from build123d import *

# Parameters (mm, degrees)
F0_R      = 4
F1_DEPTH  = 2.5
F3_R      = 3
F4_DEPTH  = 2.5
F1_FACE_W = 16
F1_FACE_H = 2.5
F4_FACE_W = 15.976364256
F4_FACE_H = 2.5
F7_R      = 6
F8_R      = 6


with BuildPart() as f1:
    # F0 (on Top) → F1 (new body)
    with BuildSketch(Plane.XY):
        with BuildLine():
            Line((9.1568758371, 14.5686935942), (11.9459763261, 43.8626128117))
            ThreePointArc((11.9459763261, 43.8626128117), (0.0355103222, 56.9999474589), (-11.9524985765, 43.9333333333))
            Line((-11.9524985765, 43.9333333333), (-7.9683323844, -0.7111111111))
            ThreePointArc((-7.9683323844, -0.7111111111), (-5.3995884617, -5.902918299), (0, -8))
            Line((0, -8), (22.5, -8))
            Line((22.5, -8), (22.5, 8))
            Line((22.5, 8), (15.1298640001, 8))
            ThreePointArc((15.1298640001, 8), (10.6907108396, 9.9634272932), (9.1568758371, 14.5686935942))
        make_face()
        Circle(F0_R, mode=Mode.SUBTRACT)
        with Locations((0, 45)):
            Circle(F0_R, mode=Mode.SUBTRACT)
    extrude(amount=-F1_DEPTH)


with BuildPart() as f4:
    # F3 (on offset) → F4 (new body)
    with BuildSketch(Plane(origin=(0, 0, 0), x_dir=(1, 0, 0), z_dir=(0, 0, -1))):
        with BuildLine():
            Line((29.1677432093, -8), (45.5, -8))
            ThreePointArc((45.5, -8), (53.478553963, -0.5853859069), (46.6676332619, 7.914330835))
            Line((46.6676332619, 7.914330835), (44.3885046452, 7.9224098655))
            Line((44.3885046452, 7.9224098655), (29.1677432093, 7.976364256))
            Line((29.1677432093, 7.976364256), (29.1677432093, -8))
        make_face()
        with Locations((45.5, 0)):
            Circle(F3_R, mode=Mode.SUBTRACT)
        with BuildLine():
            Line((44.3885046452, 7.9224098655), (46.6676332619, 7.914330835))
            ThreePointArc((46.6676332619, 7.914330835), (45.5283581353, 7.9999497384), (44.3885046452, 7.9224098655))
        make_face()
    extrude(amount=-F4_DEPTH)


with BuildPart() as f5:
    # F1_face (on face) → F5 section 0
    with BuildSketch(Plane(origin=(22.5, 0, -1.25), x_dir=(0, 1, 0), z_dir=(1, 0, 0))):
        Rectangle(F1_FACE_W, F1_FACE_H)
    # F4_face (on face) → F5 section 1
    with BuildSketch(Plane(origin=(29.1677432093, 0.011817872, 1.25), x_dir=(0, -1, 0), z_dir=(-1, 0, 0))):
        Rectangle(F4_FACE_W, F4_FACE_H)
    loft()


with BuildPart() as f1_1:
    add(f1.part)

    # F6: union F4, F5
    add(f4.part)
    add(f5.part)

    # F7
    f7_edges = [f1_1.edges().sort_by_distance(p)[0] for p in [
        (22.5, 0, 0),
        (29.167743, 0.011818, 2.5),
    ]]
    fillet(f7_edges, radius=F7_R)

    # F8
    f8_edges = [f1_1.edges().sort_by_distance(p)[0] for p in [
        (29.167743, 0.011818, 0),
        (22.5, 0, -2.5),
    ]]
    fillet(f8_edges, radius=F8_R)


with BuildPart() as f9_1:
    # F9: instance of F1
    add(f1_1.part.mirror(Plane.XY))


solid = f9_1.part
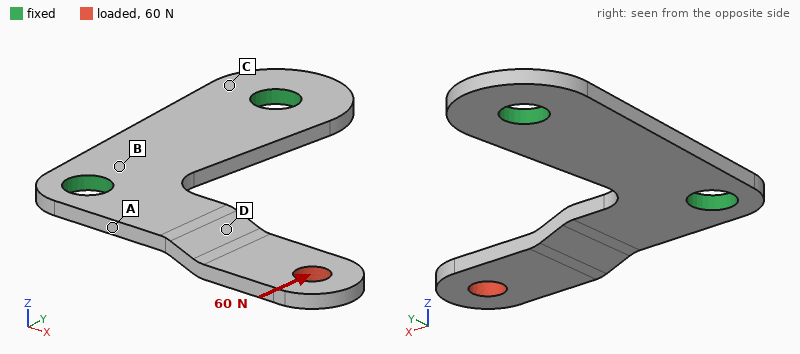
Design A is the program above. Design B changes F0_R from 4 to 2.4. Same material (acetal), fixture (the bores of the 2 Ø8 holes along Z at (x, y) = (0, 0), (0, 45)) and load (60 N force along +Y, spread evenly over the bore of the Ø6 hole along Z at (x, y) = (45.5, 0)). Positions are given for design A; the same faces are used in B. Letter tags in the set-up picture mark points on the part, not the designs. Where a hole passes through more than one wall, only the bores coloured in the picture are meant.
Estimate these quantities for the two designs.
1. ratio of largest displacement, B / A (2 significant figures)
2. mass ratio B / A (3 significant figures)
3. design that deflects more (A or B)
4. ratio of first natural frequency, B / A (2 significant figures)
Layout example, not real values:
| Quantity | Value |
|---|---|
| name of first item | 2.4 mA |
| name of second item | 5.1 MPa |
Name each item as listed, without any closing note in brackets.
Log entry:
| Quantity | Value |
|---|---|
| ratio of largest displacement, B / A | 1.1 |
| mass ratio B / A | 1.04 |
| design that deflects more | B |
| ratio of first natural frequency, B / A | 0.94 |
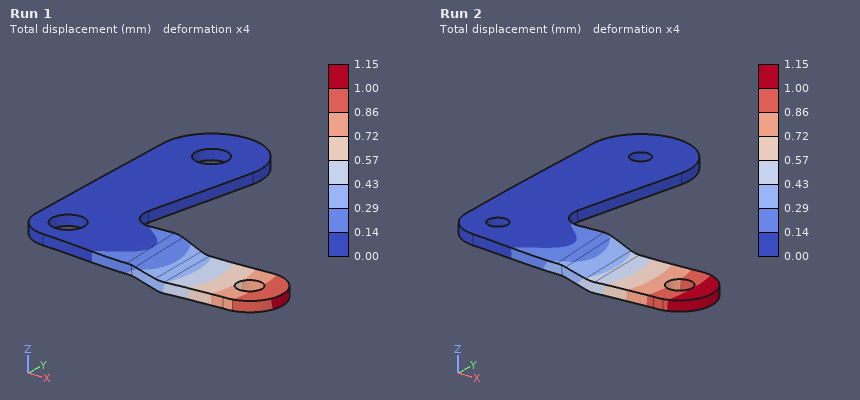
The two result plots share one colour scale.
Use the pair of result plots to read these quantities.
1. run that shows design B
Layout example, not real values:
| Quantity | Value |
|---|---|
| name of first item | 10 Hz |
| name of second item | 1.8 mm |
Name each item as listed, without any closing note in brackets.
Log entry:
| Quantity | Value |
|---|---|
| run that shows design B | Run 2 |
